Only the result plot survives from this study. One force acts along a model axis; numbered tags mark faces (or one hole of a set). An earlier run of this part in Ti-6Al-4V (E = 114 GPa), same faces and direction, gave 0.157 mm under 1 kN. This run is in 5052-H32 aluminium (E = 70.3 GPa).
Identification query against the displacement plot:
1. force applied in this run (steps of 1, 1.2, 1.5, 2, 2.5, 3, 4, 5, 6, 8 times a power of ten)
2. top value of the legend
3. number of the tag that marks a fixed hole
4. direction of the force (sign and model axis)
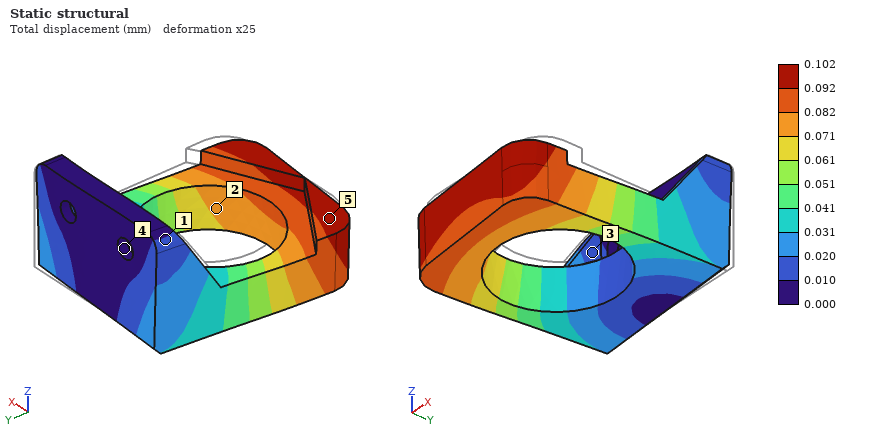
400 N
0.102 mm
4
-X
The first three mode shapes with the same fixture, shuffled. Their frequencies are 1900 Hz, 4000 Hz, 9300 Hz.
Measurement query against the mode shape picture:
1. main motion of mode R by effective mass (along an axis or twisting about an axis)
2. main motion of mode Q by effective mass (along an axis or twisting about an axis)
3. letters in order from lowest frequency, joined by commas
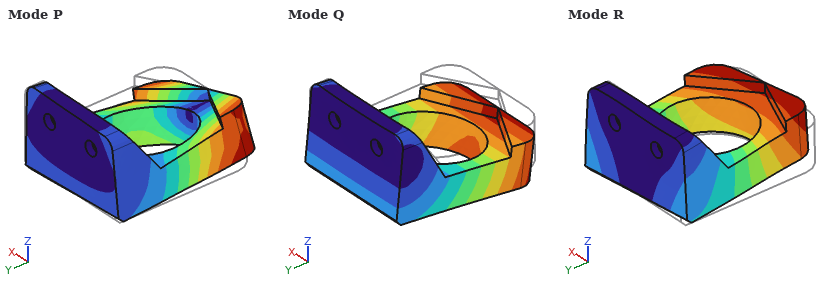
along X
along Z
Q, R, P
